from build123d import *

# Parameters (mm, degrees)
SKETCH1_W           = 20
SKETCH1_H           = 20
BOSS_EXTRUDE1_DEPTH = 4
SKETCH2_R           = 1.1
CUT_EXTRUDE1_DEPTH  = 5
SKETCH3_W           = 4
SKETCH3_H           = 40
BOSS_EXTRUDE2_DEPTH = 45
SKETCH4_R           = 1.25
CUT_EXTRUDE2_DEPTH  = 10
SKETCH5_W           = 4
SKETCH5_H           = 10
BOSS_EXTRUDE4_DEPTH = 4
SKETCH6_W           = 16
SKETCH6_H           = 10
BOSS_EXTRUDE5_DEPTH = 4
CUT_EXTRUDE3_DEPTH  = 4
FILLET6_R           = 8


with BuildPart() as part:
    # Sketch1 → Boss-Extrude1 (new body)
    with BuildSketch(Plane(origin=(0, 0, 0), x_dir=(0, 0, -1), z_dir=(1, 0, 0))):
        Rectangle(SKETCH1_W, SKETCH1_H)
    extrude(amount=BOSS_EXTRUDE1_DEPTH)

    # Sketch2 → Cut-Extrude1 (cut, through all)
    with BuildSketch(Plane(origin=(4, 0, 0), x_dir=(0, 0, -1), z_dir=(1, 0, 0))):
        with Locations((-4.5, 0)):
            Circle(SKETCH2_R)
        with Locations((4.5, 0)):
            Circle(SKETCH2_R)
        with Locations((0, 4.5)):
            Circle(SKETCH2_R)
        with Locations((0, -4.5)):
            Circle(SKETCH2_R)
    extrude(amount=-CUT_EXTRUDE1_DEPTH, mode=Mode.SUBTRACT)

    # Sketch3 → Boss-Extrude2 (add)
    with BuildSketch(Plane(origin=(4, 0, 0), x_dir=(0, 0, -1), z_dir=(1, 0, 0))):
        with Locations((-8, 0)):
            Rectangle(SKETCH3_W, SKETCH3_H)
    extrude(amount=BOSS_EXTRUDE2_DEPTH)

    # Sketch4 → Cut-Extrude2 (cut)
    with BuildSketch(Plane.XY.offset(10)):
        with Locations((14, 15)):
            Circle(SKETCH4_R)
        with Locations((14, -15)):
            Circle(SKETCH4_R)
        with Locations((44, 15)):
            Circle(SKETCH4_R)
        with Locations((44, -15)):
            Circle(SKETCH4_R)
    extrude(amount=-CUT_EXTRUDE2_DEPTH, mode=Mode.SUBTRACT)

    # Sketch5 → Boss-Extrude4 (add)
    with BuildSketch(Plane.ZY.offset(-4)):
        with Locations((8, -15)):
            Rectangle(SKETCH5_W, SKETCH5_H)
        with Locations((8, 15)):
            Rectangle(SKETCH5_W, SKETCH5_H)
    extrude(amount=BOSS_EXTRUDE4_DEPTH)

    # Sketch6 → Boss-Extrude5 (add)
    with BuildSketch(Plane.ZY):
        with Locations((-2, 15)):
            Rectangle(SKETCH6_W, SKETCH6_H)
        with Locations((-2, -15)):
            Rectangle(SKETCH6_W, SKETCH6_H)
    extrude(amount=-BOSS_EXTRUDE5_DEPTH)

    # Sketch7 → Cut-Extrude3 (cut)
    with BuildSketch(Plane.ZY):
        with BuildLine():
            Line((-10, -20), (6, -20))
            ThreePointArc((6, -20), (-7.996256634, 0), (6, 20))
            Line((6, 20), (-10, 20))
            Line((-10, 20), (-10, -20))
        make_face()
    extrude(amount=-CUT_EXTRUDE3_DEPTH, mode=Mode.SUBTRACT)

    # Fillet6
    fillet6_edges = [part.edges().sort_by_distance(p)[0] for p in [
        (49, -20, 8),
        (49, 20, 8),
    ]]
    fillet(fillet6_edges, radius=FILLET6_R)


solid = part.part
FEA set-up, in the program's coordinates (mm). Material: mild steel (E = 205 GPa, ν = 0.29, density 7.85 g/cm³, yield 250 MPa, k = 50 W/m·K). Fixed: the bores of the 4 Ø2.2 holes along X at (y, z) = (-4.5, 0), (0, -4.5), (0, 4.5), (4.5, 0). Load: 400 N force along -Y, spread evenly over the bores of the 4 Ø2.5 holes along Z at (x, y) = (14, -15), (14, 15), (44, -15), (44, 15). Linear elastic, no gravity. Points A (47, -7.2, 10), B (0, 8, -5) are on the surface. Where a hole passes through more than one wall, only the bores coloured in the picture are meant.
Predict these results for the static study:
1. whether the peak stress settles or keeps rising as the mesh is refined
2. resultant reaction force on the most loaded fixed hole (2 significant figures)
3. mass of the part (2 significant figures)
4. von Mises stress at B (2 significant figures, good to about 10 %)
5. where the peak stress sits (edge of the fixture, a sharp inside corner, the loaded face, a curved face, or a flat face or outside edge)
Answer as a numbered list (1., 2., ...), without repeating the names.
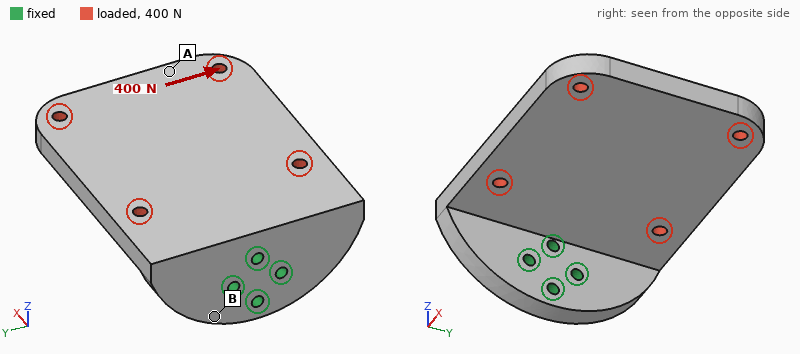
1. keeps rising
2. 570 N
3. 72 g
4. 37 MPa
5. edge of the fixture
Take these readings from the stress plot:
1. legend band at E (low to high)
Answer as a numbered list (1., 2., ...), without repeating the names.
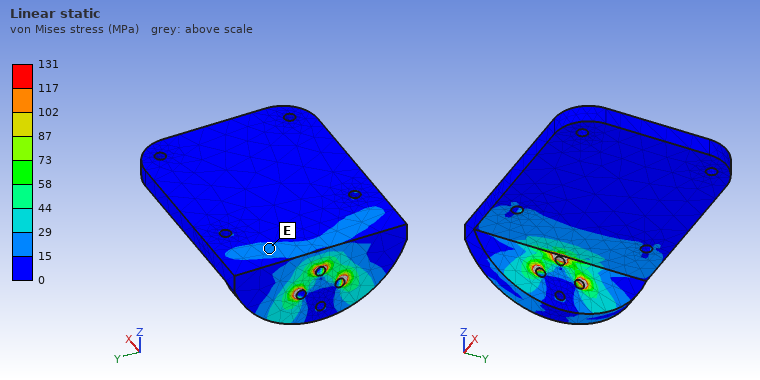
1. 15 to 29 MPa
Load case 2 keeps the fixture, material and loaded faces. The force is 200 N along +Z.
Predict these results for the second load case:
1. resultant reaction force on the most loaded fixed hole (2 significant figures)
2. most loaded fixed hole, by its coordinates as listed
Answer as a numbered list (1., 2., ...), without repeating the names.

1. 480 N
2. (0, 4.5)
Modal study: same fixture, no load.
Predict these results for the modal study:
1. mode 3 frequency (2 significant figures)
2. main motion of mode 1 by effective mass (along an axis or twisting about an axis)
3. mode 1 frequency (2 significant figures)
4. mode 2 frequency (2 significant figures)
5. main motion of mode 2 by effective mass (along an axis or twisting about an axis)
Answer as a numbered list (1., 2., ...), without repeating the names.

1. 4000 Hz
2. along Z
3. 1300 Hz
4. 2500 Hz
5. along Y
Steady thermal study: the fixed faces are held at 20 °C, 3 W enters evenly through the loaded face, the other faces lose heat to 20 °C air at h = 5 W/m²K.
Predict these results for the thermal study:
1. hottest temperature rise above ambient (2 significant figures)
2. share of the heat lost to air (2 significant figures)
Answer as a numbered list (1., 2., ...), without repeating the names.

1. 14 K
2. 6.6 %
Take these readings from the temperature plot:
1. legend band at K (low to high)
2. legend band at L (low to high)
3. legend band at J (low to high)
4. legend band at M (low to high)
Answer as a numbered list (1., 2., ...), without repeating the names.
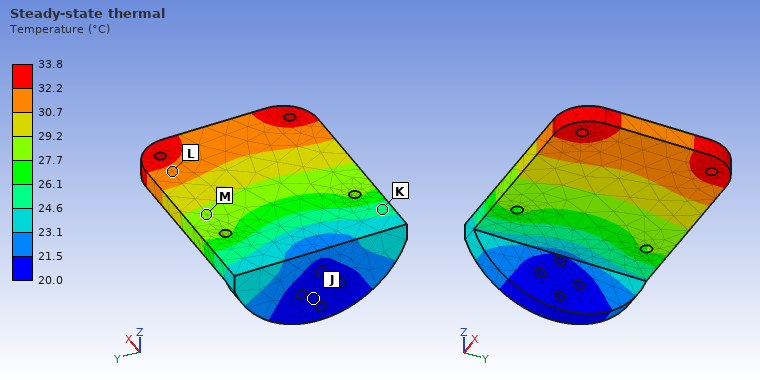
1. 24.6 to 26.1 °C
2. 30.7 to 32.2 °C
3. 20.0 to 21.5 °C
4. 27.7 to 29.2 °C
